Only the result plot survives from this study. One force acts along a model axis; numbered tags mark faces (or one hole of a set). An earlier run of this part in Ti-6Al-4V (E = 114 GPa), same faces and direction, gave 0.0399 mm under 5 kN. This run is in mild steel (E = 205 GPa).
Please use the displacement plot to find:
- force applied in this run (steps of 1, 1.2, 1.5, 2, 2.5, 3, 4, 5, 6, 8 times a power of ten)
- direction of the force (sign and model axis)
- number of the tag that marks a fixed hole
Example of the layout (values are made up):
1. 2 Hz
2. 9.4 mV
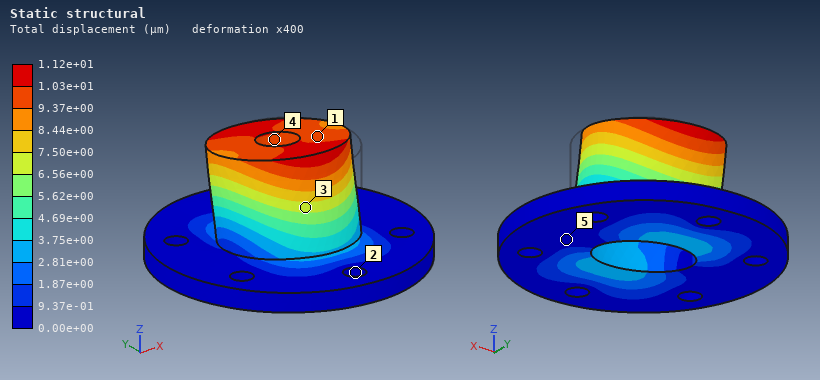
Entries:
1. 2.5 kN
2. +Y
3. 2
